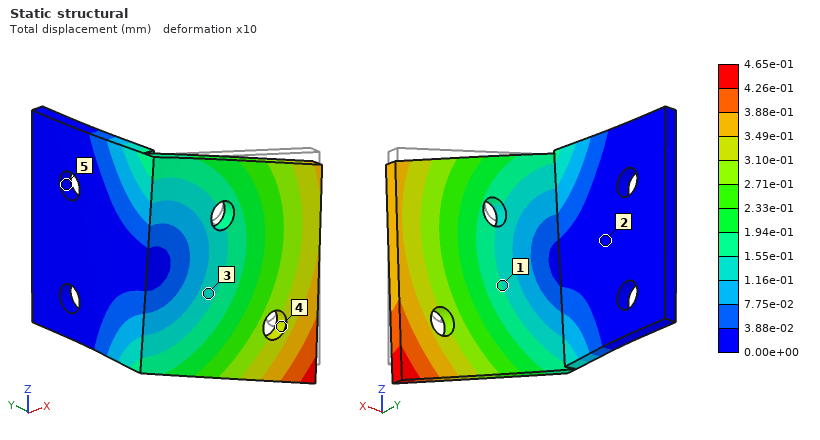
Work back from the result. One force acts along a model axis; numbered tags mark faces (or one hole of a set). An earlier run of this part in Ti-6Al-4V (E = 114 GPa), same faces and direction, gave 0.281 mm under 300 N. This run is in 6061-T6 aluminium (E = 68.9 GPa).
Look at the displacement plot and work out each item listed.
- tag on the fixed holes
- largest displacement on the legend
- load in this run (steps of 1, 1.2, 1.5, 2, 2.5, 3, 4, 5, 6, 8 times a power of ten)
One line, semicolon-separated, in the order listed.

5; 4.65e-01 mm; 300 N
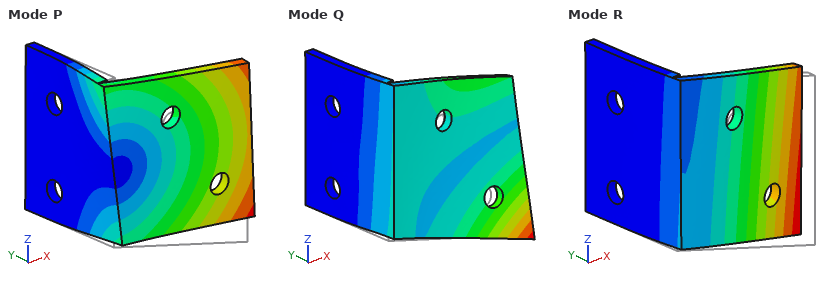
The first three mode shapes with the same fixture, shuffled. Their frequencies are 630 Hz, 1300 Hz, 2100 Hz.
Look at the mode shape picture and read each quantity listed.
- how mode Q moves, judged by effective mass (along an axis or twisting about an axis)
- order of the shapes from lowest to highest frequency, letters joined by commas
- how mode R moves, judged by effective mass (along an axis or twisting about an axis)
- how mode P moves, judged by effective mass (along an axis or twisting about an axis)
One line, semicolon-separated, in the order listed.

along X; R, P, Q; along Y; along Z
